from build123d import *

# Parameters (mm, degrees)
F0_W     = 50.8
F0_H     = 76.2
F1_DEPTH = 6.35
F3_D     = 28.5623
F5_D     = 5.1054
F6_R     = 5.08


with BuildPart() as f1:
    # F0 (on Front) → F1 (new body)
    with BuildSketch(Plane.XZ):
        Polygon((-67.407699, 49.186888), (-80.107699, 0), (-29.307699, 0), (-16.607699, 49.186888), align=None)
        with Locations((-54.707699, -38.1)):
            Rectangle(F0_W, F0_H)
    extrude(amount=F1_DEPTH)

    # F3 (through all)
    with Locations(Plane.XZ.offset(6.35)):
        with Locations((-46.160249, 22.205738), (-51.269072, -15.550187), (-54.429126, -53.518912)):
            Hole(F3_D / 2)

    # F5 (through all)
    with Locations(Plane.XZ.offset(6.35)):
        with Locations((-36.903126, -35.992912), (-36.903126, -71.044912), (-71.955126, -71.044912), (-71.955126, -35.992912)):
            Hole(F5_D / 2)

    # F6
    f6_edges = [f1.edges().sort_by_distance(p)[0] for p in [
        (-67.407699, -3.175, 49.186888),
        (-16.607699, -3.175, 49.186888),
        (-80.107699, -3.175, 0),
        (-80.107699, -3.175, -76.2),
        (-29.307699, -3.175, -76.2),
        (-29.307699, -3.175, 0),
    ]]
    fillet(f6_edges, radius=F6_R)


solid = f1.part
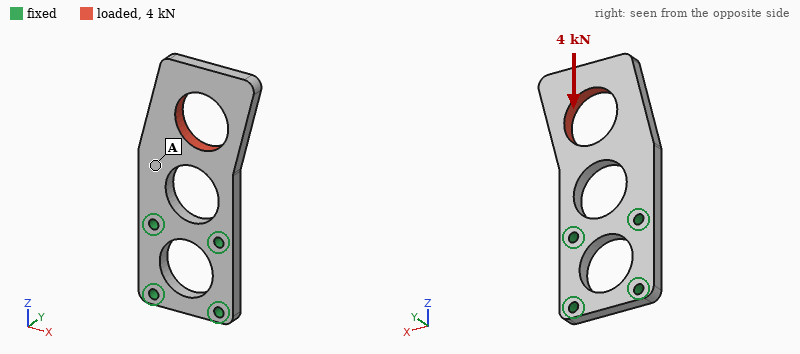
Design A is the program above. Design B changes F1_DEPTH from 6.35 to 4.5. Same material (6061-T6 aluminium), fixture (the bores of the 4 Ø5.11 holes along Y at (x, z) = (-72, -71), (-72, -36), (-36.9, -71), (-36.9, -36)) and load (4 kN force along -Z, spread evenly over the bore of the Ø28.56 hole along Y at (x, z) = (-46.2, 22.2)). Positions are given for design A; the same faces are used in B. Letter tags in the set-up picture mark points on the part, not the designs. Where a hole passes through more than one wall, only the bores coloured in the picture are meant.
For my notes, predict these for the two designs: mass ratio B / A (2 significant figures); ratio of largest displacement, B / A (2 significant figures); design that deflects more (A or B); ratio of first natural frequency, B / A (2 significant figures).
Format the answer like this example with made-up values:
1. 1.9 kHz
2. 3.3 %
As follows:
1. 0.71
2. 1.4
3. B
4. 0.72
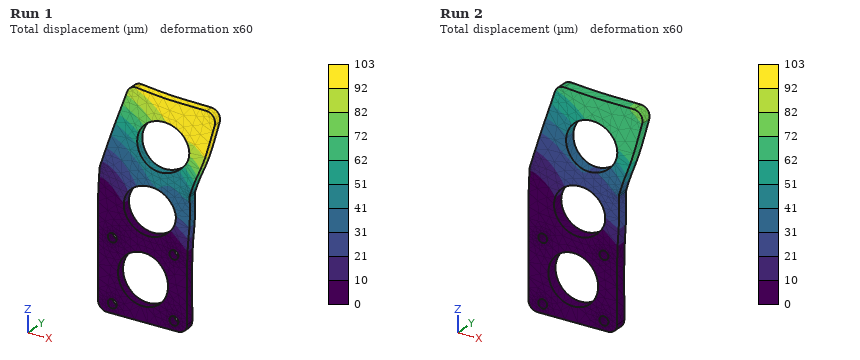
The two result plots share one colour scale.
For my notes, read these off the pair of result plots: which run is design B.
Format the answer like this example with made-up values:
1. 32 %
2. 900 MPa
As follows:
1. Run 1
